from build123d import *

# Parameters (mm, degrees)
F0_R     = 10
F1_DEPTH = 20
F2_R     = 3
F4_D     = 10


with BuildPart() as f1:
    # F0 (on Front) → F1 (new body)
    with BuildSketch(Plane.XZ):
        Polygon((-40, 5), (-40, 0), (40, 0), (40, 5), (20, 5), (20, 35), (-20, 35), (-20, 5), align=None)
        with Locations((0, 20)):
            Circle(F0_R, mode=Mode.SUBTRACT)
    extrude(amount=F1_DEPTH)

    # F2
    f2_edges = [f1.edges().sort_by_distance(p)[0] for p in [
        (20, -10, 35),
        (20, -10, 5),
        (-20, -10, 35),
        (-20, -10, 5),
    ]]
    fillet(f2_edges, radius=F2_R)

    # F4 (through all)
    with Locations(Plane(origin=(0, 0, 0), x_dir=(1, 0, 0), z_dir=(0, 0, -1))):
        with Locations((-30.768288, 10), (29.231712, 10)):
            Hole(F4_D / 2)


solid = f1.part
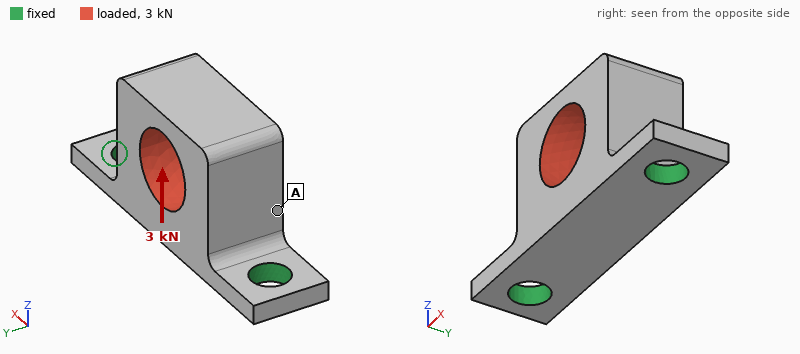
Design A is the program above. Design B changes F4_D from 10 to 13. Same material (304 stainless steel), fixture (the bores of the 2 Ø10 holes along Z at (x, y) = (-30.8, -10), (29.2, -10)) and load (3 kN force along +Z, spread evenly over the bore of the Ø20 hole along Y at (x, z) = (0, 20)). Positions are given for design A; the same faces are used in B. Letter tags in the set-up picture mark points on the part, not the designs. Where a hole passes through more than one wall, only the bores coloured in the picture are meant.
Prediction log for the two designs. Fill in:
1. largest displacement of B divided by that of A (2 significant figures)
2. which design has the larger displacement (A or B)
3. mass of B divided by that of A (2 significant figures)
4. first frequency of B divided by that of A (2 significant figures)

0.74
A
0.98
1.2
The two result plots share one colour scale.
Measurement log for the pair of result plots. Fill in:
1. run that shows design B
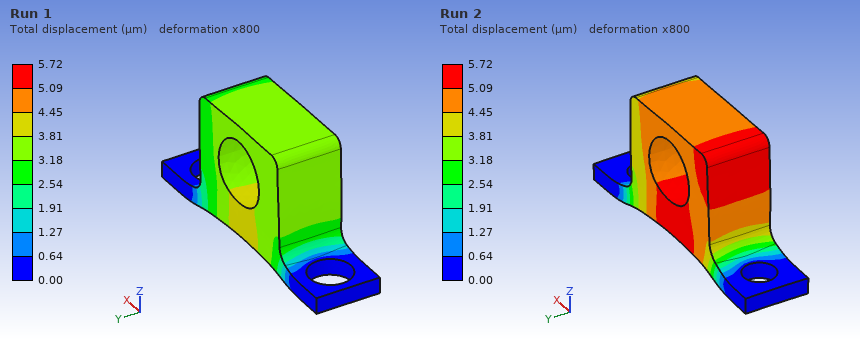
Run 1
